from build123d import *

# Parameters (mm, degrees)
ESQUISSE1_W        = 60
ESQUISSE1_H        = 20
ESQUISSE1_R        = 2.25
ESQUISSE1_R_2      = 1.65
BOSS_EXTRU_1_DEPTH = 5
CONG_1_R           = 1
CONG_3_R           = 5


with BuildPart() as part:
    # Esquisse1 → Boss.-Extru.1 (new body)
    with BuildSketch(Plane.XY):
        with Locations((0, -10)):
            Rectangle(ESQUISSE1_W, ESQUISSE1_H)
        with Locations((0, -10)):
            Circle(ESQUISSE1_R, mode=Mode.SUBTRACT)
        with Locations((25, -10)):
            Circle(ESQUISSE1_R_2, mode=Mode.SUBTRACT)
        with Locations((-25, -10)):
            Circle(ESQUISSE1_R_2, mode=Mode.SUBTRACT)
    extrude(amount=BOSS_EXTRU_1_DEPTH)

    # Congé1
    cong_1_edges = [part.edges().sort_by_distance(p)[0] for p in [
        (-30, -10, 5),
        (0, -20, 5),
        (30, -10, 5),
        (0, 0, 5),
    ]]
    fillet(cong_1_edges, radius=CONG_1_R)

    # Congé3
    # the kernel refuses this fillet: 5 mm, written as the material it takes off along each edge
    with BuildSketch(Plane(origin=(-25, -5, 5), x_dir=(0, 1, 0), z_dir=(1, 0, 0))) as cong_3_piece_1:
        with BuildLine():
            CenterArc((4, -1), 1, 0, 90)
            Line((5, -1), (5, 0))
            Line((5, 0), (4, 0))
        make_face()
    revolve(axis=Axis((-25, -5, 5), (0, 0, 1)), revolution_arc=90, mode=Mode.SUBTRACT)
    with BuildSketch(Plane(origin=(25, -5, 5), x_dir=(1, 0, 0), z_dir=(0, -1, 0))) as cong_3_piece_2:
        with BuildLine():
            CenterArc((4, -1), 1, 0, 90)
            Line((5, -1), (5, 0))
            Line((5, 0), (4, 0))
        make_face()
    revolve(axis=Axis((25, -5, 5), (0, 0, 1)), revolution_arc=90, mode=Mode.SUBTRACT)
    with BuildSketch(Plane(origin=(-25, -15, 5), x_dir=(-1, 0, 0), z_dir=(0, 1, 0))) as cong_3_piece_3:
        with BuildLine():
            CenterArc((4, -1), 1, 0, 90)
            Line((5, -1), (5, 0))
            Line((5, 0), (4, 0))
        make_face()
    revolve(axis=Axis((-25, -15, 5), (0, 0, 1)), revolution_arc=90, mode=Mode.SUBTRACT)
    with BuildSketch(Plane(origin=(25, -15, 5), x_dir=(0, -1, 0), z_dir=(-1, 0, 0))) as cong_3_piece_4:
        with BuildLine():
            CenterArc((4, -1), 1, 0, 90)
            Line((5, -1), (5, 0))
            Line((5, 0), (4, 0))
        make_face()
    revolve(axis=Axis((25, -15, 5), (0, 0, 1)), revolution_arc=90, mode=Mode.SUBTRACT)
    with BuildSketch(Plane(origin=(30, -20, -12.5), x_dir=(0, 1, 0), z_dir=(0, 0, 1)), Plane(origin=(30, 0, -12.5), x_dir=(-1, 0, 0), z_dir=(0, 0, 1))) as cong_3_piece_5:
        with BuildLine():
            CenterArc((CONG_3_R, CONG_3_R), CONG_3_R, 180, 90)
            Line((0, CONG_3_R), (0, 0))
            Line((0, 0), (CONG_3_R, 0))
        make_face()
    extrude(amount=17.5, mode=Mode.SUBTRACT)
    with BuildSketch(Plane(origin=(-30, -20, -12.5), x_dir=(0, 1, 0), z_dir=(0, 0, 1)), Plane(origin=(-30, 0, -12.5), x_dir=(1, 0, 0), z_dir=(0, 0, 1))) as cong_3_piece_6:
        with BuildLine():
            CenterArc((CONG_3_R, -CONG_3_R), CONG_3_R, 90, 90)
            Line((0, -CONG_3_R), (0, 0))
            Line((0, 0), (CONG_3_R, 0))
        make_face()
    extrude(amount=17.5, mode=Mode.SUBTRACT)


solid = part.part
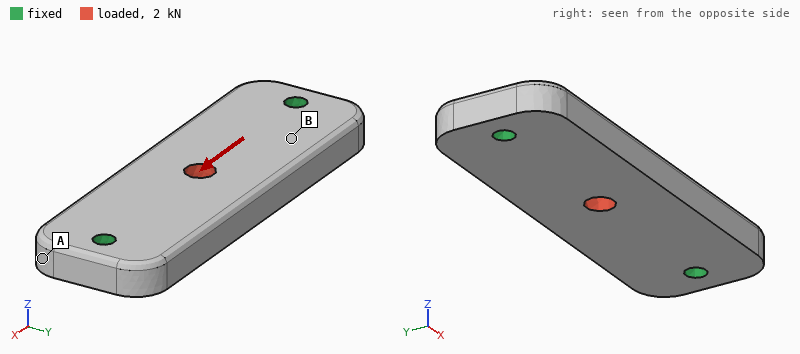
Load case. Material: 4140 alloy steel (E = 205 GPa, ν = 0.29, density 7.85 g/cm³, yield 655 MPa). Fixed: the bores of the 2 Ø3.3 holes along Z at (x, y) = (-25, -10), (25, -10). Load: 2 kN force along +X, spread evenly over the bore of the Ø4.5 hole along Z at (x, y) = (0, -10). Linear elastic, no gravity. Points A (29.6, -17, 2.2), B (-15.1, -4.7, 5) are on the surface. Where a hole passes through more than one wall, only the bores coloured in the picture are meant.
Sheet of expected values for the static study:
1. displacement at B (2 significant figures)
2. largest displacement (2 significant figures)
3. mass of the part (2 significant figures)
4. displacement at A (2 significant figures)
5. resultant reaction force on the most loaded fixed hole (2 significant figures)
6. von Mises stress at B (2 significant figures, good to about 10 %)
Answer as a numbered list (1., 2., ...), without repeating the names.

1. 0.85 µm
2. 2.0 µm
3. 45 g
4. 0.58 µm
5. 1.0 kN
6. 11 MPa
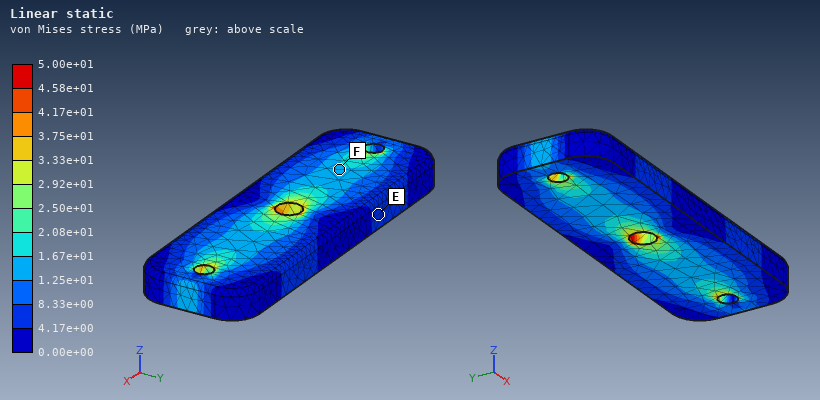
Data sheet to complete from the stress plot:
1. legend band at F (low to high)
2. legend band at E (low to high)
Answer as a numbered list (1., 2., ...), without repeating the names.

1. 1.25e+01 to 1.67e+01 MPa
2. 4.17e+00 to 8.33e+00 MPa
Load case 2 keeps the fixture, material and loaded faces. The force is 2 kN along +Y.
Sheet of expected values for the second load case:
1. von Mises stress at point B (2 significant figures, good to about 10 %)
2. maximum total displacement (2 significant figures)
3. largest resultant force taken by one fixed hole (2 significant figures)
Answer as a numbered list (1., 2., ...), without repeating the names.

1. 21 MPa
2. 9.3 µm
3. 1.0 kN
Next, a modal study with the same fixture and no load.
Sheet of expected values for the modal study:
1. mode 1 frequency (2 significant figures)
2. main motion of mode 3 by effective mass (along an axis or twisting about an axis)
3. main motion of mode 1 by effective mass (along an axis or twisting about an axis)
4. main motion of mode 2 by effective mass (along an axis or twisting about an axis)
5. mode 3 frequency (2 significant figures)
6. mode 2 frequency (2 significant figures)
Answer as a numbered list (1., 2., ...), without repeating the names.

1. 9000 Hz
2. along Y
3. along Z
4. twisting about X
5. 17 kHz
6. 14 kHz
